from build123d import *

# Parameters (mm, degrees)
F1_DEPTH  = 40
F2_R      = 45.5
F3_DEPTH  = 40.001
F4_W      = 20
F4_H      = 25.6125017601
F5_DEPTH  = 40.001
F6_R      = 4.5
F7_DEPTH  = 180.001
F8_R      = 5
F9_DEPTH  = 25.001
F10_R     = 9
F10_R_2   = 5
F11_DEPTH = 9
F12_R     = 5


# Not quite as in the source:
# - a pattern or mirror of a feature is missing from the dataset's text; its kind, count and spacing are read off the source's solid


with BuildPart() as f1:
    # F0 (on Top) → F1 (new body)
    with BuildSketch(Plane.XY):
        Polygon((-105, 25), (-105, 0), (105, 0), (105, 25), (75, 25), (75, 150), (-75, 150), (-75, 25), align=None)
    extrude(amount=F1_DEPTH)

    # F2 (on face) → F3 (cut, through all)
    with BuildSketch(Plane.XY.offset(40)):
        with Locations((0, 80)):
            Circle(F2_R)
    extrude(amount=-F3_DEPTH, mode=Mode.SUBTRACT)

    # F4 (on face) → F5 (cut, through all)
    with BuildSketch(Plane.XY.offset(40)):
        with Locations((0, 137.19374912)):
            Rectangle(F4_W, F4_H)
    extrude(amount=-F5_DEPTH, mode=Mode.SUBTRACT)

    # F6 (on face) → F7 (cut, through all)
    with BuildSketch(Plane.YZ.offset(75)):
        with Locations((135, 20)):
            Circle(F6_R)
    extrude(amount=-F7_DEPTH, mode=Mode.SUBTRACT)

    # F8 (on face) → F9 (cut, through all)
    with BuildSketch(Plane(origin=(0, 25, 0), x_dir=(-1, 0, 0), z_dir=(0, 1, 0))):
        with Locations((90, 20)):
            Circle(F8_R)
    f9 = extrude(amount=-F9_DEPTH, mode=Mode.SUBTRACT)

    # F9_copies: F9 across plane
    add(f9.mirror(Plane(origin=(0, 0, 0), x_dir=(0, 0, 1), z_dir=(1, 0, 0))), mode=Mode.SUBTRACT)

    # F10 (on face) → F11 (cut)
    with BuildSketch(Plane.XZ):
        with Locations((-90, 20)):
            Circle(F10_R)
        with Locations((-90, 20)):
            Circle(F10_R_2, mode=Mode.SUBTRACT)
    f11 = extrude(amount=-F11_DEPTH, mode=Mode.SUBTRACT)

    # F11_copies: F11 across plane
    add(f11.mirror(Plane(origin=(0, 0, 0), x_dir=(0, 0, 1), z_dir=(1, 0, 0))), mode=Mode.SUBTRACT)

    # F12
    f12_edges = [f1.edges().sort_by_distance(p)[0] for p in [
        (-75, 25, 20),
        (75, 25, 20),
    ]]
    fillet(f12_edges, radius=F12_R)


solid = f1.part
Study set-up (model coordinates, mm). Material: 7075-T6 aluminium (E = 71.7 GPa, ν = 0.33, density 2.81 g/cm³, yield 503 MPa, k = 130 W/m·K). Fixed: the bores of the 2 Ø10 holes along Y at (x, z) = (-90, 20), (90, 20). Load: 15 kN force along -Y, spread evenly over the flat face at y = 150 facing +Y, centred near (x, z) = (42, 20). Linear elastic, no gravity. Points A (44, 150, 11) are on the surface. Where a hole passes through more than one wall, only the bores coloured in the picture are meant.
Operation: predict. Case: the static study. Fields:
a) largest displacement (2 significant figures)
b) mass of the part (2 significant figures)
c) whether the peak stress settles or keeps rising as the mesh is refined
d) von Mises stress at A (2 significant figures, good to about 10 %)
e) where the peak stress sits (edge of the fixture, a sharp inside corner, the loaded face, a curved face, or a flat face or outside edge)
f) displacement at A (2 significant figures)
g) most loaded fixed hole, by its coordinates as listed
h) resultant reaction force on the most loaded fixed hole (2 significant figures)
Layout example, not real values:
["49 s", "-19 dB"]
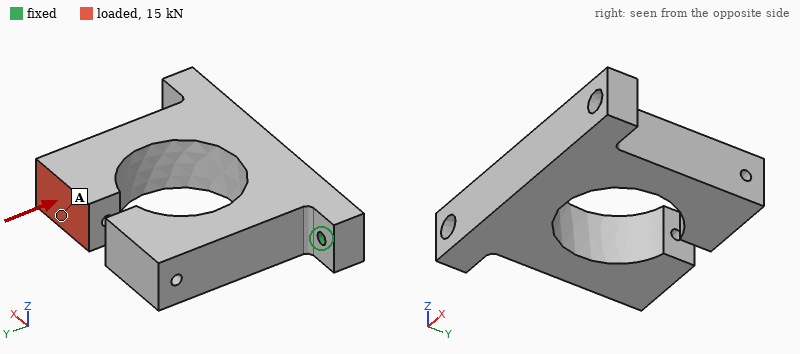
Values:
["0.34 mm", "1.9 kg", "keeps rising", "10 MPa", "edge of the fixture", "0.29 mm", "(90, 20)", "12 kN"]
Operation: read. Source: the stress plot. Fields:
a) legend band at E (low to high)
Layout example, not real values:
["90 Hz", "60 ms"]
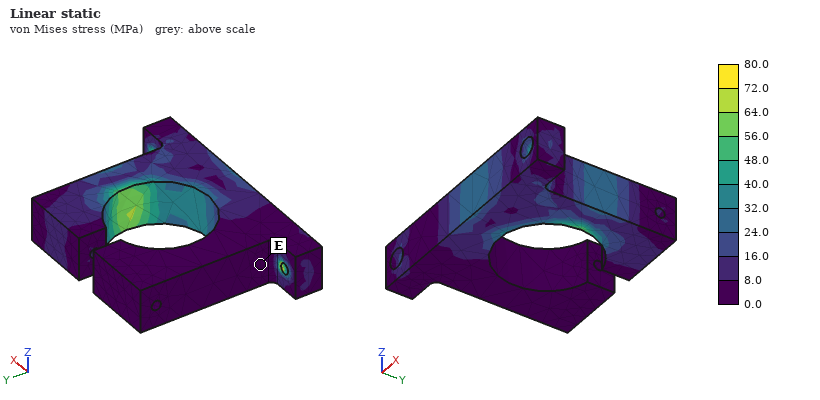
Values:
["0.0 to 8.0 MPa"]
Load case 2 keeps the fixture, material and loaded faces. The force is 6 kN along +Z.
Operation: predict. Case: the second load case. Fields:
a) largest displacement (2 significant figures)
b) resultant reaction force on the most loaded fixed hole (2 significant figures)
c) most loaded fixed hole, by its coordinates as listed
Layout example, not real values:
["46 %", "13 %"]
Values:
["1.1 mm", "4.6 kN", "(90, 20)"]
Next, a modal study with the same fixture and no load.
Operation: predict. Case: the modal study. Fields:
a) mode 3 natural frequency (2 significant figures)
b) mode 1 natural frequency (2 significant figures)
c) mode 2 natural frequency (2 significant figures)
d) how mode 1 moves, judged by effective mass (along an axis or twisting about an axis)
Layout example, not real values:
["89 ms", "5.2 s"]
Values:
["1000 Hz", "640 Hz", "1000 Hz", "along Z"]
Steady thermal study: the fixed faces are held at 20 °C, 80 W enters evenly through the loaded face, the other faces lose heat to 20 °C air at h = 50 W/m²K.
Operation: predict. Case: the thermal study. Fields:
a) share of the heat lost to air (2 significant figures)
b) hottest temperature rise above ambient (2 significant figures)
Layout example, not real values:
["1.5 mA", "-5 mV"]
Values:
["50 %", "45 K"]
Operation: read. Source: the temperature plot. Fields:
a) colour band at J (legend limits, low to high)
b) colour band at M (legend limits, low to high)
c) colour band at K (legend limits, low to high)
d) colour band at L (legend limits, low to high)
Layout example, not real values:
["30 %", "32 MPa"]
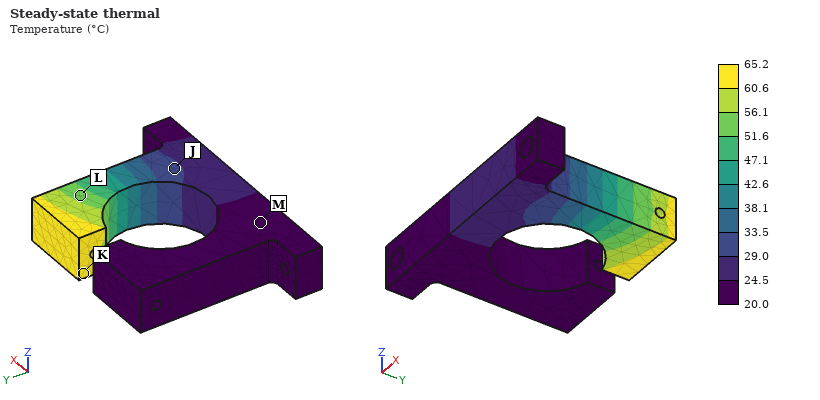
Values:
["29.0 to 33.5 °C", "20.0 to 24.5 °C", "60.6 to 65.2 °C", "51.6 to 56.1 °C"]
